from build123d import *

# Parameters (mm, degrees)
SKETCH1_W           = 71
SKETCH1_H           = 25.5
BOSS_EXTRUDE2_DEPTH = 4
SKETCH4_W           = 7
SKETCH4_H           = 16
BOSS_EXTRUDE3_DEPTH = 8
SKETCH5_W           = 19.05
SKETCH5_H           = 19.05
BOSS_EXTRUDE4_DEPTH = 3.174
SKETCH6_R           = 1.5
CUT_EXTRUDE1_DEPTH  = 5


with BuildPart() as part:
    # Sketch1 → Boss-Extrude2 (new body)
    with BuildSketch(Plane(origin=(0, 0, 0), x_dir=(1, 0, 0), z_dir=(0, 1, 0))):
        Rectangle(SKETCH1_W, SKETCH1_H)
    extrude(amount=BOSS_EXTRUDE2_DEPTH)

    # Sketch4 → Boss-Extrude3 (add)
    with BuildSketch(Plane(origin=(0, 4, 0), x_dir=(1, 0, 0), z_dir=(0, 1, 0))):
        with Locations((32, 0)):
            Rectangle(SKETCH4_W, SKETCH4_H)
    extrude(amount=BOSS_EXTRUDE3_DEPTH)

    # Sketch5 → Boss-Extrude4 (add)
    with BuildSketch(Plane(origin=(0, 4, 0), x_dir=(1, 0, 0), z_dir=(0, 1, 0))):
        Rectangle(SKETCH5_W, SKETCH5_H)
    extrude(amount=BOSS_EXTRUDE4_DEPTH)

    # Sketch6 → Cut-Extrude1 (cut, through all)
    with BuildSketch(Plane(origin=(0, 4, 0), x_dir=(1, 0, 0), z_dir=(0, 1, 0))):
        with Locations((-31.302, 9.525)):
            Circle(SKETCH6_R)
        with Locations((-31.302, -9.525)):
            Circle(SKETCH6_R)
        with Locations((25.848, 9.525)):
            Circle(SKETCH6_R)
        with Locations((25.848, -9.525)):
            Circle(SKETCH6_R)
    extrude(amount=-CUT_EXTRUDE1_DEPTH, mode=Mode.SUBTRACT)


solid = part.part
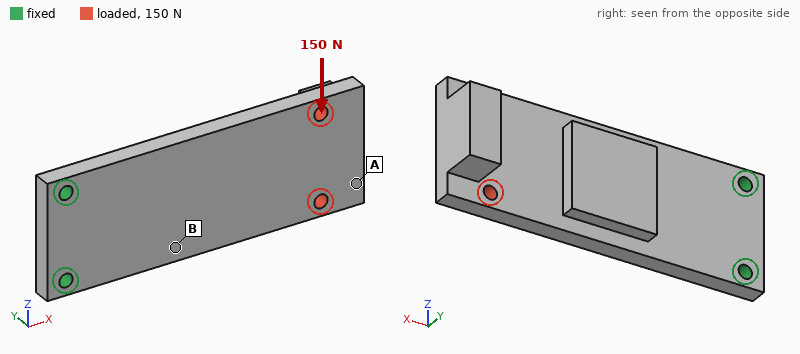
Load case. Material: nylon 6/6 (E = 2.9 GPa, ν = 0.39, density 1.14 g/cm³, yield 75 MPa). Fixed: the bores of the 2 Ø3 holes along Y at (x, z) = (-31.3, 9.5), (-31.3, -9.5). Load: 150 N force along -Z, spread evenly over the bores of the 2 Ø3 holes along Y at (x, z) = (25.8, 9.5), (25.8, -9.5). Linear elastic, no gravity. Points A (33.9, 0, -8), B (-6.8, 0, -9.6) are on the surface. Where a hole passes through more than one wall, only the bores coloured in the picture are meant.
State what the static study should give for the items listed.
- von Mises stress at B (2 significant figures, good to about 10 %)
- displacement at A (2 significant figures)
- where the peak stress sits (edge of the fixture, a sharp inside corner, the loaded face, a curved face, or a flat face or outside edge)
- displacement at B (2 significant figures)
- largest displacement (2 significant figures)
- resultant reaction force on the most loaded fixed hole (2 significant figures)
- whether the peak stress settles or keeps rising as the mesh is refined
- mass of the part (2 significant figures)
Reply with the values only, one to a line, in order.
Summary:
8.6 MPa
0.79 mm
edge of the fixture
0.20 mm
0.82 mm
440 N
keeps rising
10 g
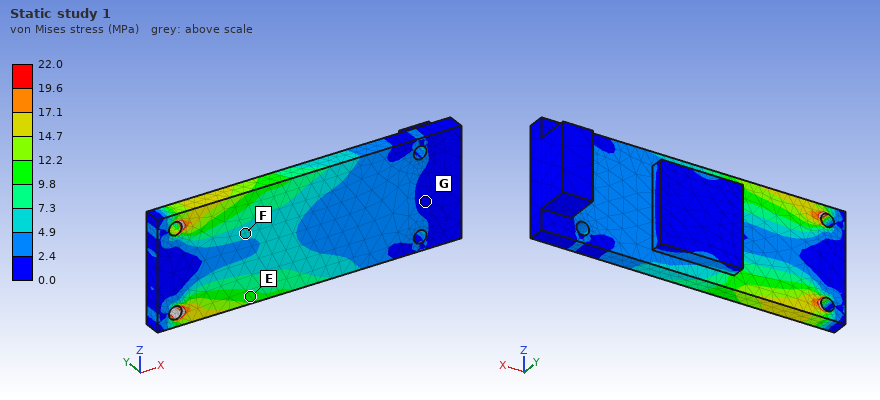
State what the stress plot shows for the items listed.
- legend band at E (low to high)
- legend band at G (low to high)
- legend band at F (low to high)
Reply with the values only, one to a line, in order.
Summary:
9.8 to 12.2 MPa
0.0 to 2.4 MPa
4.9 to 7.3 MPa
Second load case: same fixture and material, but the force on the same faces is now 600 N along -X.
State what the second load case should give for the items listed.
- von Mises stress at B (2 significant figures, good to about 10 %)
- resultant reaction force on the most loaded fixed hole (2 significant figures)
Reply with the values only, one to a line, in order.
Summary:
7.3 MPa
310 N
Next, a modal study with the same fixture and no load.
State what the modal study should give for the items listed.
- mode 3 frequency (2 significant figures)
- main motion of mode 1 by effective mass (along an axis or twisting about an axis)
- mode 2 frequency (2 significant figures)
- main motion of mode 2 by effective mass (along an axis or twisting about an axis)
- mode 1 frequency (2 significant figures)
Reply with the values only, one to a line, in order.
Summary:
1300 Hz
along Y
1100 Hz
along Z
200 Hz
